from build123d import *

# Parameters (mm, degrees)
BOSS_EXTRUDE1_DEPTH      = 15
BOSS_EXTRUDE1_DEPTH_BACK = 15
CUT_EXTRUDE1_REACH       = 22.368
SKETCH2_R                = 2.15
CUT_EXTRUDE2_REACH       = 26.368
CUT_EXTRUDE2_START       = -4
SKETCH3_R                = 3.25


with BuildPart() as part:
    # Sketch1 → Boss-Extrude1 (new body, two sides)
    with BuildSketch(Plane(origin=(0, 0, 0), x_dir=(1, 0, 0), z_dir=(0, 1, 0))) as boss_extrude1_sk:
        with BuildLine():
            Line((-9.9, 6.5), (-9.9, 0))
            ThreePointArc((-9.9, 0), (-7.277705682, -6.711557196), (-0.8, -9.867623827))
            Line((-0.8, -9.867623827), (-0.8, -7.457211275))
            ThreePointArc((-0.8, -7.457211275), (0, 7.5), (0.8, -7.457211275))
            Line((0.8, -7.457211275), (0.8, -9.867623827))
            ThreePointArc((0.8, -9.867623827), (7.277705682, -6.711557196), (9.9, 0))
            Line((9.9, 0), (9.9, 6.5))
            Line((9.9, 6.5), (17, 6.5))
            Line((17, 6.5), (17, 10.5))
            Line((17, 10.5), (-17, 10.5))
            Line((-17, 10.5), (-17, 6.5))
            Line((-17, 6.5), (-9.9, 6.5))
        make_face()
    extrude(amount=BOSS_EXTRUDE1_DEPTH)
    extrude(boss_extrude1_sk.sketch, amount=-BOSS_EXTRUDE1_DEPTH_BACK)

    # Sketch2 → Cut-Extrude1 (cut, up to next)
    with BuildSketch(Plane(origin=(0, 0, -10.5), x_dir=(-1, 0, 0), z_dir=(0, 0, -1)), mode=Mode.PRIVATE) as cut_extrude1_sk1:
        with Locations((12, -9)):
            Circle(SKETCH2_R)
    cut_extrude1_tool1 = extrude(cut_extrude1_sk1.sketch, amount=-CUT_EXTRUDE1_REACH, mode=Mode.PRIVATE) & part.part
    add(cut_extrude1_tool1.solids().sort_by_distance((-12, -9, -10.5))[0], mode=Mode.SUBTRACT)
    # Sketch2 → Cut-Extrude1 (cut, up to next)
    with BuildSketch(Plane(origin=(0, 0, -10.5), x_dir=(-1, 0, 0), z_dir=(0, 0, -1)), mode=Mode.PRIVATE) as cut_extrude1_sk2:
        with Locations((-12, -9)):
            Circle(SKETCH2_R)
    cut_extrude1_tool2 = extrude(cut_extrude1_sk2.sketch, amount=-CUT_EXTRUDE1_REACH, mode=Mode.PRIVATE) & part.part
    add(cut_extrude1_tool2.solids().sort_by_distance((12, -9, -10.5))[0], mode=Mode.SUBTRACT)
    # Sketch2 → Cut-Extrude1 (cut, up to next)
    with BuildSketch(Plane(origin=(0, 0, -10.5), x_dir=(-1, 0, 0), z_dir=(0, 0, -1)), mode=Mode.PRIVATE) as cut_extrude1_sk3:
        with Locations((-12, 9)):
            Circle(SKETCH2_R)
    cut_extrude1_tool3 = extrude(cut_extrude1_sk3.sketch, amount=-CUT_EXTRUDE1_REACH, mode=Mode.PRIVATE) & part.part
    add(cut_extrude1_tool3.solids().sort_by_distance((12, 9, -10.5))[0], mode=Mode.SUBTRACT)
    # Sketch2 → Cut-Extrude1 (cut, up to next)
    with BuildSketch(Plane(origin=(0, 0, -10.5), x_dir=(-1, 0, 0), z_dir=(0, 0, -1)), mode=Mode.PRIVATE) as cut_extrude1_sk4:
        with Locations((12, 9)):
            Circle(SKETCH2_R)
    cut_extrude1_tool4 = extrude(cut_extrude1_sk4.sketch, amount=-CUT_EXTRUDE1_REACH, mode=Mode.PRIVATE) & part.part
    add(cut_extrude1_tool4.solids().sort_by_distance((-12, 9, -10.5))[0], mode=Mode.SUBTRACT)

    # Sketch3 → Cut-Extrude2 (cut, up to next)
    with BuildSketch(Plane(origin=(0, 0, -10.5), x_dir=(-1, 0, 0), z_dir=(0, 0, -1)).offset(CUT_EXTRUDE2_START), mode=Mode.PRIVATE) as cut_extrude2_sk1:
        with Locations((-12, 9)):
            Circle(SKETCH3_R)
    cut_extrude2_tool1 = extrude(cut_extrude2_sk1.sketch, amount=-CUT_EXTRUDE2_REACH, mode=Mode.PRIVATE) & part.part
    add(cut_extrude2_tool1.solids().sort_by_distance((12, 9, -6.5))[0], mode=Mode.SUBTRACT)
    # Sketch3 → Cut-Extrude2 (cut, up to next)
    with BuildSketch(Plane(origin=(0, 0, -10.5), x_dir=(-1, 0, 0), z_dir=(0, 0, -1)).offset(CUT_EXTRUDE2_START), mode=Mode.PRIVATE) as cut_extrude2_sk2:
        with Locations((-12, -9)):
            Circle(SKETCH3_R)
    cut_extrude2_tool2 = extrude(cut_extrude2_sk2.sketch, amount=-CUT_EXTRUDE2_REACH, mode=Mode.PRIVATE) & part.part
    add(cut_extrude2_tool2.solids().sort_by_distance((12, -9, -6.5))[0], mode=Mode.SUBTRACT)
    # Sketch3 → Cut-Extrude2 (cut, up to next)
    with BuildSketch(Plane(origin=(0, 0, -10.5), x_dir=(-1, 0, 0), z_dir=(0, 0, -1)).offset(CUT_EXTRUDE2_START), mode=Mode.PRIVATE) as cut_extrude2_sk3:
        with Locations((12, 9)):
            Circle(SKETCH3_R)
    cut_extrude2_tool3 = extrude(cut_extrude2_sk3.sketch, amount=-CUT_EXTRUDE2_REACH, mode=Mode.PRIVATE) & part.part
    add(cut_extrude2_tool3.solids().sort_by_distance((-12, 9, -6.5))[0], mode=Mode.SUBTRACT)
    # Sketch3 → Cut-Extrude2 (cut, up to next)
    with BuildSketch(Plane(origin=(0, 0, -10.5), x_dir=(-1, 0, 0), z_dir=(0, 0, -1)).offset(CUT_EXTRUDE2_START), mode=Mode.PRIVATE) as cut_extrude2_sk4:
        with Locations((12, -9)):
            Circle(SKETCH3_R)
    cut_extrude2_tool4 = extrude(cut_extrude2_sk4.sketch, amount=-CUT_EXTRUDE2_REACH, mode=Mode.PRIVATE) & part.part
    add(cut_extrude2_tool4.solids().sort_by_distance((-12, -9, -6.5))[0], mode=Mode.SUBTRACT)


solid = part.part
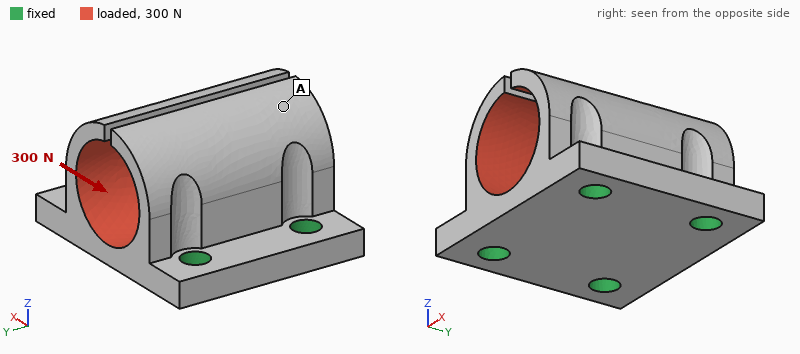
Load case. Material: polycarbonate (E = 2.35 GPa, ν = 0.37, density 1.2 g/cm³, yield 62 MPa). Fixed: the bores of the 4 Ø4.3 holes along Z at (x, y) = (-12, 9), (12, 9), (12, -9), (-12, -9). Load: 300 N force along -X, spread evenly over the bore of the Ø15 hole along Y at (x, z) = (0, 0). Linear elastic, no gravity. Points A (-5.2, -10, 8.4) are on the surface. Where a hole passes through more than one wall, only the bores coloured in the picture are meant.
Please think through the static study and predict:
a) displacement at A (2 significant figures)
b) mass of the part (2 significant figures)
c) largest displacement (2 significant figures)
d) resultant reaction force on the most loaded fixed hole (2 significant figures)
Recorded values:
0.43 mm
8.1 g
0.56 mm
90 N
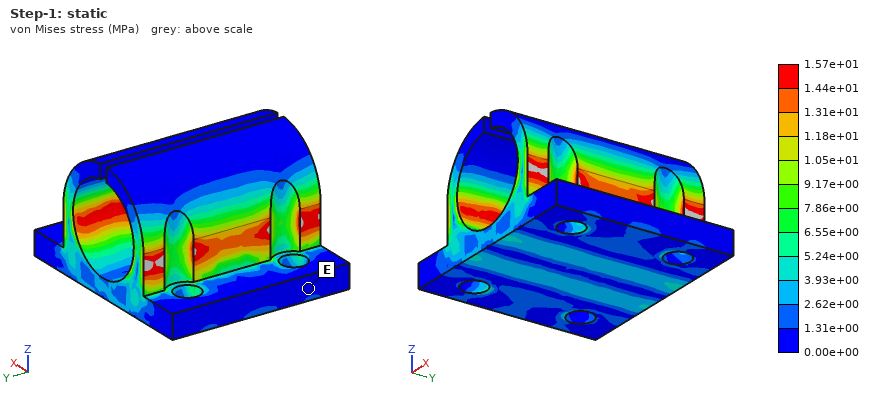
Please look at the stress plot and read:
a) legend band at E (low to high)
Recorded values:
0.00e+00 to 1.31e+00 MPa
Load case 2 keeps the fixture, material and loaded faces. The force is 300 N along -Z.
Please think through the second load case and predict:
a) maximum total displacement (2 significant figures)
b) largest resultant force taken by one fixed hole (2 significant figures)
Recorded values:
0.45 mm
76 N
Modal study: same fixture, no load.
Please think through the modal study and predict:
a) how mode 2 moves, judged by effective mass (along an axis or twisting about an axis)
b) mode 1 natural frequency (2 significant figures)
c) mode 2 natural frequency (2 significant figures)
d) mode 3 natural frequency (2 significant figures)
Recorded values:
along X
1800 Hz
1900 Hz
2800 Hz
